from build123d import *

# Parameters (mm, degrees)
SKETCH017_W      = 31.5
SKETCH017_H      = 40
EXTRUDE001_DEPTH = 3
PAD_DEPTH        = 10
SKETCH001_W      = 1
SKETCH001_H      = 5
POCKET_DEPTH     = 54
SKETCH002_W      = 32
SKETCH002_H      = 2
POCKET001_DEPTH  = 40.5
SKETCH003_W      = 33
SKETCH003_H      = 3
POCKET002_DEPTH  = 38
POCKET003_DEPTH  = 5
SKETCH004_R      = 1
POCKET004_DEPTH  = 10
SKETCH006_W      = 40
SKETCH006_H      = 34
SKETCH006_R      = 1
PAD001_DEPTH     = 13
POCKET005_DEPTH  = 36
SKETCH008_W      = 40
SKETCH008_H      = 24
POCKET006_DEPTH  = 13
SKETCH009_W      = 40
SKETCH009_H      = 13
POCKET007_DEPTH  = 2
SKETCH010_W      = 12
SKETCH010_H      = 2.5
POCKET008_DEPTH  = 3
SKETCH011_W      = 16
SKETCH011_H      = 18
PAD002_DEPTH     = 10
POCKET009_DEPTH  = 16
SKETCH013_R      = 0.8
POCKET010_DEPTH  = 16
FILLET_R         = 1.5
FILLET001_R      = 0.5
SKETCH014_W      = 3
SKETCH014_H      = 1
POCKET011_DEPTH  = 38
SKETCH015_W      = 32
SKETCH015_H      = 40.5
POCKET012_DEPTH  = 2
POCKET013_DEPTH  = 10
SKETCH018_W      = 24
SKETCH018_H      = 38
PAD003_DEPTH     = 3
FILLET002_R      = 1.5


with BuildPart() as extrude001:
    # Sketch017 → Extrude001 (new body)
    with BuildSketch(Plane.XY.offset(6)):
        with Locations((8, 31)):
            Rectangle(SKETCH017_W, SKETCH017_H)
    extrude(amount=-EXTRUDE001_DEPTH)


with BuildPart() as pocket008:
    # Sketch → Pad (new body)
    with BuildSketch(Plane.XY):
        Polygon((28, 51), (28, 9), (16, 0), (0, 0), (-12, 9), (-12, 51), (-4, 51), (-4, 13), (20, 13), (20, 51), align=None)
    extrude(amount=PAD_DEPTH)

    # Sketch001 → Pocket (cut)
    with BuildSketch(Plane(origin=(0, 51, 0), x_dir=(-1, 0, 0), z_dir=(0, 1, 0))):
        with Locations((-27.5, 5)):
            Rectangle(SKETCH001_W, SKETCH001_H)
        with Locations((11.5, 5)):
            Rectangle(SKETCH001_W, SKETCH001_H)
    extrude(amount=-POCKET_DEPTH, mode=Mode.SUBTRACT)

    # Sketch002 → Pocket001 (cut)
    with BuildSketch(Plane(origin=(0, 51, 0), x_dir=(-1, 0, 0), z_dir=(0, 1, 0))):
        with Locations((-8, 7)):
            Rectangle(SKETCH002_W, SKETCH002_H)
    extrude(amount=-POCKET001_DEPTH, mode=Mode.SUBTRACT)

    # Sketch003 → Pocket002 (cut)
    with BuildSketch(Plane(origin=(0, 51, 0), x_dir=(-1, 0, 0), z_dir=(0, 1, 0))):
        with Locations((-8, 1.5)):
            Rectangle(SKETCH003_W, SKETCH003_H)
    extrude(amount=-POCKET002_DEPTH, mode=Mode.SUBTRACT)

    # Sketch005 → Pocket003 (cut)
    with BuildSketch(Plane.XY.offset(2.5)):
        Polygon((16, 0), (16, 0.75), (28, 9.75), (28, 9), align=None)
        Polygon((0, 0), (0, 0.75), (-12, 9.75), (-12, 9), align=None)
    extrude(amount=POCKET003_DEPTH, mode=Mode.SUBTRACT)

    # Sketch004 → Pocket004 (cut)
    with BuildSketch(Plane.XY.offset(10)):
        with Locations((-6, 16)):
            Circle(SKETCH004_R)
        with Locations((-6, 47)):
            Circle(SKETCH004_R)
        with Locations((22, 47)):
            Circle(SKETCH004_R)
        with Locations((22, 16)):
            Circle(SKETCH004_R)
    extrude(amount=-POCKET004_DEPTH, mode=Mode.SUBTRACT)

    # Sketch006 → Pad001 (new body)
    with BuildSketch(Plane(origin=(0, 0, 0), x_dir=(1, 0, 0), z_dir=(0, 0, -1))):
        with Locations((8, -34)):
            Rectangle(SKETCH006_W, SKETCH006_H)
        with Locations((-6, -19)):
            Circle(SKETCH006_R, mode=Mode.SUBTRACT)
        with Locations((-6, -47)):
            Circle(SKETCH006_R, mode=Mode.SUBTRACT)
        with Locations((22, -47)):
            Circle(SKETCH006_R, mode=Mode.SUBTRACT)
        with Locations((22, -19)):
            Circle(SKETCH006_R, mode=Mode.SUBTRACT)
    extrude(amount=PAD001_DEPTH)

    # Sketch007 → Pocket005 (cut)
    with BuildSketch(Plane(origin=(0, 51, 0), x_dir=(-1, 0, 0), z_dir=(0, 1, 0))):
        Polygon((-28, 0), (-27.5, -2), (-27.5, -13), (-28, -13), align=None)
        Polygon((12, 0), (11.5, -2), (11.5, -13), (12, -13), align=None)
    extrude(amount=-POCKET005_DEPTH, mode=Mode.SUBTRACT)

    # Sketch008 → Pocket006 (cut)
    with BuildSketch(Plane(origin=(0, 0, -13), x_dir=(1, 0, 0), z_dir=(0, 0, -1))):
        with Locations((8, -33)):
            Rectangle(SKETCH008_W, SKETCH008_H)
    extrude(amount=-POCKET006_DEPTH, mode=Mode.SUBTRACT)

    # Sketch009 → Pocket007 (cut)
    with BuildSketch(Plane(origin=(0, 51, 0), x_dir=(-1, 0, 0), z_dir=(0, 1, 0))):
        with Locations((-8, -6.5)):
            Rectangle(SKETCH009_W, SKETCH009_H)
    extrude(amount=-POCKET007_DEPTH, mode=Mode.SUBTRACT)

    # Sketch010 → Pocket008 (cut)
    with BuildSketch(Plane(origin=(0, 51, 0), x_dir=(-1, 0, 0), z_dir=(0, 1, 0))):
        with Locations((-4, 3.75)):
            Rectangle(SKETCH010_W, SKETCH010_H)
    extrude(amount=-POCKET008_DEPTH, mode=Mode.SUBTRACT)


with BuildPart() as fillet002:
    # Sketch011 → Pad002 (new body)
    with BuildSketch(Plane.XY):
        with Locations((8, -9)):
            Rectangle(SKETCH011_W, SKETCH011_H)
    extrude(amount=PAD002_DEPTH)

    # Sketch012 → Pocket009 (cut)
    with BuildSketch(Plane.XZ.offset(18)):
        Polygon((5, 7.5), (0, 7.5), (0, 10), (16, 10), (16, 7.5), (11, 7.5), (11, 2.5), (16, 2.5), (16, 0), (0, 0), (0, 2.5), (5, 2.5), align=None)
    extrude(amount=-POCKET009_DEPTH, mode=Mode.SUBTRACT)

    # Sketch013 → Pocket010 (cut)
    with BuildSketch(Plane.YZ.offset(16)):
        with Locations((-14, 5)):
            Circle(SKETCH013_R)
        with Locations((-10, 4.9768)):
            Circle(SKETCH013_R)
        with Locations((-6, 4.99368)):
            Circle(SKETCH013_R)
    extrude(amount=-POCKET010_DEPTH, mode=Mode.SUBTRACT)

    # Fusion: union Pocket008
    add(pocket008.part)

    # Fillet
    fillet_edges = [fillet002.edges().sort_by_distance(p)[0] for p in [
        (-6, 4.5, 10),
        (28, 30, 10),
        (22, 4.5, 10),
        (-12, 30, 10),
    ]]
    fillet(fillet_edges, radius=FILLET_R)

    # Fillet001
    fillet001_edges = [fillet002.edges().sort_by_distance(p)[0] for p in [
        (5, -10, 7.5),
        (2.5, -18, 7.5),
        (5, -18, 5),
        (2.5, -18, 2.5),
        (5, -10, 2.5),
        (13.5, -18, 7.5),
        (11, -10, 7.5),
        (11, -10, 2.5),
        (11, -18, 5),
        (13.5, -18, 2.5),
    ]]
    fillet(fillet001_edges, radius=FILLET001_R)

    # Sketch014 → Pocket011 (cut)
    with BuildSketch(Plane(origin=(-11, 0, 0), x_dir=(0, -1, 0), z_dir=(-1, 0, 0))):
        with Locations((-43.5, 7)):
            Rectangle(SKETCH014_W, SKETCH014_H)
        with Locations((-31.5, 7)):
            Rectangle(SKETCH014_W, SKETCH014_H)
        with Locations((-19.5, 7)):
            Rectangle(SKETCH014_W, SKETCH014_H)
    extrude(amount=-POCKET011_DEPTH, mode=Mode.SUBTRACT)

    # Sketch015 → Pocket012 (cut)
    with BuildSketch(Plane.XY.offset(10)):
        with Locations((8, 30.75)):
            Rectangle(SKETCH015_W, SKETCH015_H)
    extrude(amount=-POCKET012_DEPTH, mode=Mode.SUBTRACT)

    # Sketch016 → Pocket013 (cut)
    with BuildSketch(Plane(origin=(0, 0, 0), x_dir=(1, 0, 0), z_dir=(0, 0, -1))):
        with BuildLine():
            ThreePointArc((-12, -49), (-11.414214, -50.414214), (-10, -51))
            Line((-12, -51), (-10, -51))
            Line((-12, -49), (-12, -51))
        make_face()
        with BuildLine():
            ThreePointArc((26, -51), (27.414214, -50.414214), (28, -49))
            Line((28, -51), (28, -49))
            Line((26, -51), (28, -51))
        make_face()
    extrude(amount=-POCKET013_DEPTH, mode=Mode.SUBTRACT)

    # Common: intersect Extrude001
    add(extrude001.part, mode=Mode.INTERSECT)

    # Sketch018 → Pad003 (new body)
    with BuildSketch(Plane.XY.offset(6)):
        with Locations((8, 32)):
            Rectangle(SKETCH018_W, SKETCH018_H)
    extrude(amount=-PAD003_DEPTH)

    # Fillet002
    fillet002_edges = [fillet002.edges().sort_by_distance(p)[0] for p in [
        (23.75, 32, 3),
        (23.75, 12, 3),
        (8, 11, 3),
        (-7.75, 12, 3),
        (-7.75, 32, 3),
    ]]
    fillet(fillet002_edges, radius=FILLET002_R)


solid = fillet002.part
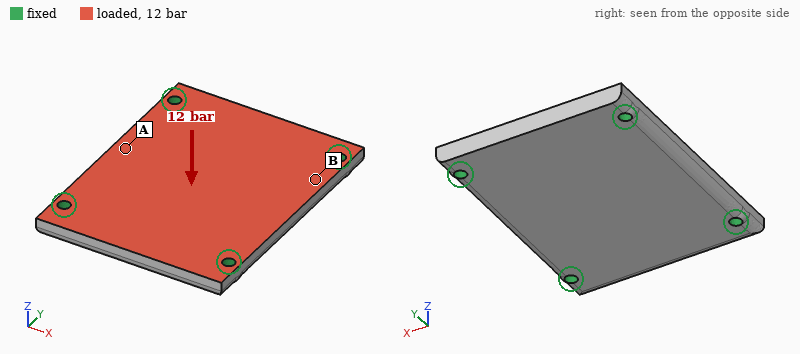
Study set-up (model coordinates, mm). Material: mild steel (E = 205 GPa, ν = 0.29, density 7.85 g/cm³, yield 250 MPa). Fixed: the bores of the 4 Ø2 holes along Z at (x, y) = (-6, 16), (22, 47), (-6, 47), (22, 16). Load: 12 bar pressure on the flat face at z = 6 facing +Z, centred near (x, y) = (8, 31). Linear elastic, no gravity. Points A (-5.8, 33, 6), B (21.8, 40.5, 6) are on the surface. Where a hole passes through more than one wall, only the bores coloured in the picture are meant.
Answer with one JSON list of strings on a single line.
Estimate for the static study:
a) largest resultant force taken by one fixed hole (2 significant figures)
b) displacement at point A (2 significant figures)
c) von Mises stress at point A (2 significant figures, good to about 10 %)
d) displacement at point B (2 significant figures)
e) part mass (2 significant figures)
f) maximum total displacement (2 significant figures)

["380 N", "11 µm", "45 MPa", "5.3 µm", "29 g", "16 µm"]
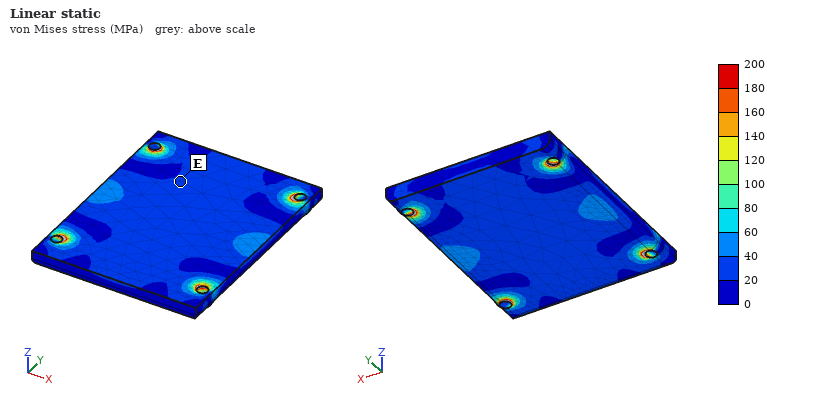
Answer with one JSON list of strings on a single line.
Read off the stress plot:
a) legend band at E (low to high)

["20 to 40 MPa"]
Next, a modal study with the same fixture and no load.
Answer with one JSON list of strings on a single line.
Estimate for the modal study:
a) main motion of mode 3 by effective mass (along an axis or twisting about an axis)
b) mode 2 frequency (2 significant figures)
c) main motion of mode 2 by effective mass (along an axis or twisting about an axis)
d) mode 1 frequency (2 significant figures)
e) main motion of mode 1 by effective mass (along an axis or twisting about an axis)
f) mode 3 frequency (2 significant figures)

["twisting about X", "18 kHz", "twisting about Y", "11 kHz", "along Z", "19 kHz"]
